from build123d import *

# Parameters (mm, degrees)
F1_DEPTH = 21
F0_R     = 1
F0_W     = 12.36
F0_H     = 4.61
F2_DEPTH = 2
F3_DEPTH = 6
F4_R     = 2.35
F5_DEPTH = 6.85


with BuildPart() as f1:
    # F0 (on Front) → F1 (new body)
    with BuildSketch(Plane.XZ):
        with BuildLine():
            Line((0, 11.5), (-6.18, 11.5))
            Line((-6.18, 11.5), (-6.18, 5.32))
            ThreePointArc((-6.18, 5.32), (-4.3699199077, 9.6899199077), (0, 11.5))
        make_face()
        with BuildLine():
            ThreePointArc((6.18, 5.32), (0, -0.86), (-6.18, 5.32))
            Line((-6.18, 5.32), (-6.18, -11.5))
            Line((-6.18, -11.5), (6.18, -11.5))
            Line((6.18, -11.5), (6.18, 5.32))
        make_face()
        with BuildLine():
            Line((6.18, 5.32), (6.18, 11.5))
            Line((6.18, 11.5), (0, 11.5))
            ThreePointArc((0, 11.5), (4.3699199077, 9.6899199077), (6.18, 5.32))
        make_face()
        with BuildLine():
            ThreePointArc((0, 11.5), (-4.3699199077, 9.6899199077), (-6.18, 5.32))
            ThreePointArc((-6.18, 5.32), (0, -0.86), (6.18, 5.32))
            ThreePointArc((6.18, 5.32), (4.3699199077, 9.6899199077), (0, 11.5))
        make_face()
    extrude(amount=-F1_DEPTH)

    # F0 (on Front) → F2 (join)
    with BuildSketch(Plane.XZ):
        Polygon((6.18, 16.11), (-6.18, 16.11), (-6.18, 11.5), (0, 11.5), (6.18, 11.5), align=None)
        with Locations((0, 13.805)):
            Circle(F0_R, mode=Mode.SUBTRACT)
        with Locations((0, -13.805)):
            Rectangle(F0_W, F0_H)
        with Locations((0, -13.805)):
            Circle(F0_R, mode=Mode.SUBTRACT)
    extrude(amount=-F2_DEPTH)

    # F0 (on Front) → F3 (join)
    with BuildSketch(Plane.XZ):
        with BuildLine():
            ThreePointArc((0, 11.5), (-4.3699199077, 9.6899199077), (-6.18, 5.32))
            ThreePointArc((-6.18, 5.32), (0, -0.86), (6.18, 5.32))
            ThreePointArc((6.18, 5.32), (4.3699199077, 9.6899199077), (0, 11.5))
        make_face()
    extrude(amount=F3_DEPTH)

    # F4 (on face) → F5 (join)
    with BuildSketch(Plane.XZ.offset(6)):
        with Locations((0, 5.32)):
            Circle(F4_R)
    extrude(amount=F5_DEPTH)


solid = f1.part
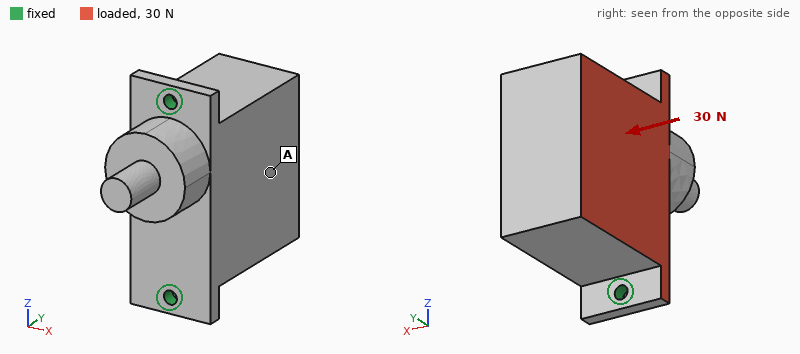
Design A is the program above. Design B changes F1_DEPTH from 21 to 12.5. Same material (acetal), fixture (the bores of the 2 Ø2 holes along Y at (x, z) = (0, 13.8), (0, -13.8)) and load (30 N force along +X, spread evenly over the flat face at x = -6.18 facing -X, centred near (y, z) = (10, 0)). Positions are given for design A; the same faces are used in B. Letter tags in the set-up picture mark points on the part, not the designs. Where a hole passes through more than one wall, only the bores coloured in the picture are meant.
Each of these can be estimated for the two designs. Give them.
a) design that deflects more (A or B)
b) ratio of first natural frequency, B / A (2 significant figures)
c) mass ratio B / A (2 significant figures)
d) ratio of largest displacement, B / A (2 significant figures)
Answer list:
A
2.0
0.66
0.35
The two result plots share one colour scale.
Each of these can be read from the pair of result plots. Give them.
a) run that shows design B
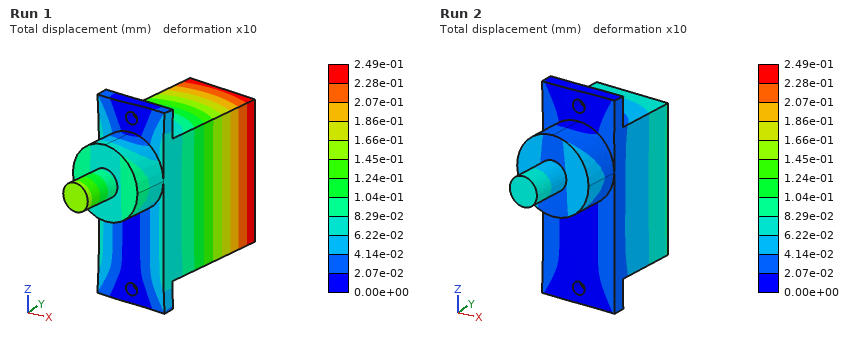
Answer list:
Run 2
